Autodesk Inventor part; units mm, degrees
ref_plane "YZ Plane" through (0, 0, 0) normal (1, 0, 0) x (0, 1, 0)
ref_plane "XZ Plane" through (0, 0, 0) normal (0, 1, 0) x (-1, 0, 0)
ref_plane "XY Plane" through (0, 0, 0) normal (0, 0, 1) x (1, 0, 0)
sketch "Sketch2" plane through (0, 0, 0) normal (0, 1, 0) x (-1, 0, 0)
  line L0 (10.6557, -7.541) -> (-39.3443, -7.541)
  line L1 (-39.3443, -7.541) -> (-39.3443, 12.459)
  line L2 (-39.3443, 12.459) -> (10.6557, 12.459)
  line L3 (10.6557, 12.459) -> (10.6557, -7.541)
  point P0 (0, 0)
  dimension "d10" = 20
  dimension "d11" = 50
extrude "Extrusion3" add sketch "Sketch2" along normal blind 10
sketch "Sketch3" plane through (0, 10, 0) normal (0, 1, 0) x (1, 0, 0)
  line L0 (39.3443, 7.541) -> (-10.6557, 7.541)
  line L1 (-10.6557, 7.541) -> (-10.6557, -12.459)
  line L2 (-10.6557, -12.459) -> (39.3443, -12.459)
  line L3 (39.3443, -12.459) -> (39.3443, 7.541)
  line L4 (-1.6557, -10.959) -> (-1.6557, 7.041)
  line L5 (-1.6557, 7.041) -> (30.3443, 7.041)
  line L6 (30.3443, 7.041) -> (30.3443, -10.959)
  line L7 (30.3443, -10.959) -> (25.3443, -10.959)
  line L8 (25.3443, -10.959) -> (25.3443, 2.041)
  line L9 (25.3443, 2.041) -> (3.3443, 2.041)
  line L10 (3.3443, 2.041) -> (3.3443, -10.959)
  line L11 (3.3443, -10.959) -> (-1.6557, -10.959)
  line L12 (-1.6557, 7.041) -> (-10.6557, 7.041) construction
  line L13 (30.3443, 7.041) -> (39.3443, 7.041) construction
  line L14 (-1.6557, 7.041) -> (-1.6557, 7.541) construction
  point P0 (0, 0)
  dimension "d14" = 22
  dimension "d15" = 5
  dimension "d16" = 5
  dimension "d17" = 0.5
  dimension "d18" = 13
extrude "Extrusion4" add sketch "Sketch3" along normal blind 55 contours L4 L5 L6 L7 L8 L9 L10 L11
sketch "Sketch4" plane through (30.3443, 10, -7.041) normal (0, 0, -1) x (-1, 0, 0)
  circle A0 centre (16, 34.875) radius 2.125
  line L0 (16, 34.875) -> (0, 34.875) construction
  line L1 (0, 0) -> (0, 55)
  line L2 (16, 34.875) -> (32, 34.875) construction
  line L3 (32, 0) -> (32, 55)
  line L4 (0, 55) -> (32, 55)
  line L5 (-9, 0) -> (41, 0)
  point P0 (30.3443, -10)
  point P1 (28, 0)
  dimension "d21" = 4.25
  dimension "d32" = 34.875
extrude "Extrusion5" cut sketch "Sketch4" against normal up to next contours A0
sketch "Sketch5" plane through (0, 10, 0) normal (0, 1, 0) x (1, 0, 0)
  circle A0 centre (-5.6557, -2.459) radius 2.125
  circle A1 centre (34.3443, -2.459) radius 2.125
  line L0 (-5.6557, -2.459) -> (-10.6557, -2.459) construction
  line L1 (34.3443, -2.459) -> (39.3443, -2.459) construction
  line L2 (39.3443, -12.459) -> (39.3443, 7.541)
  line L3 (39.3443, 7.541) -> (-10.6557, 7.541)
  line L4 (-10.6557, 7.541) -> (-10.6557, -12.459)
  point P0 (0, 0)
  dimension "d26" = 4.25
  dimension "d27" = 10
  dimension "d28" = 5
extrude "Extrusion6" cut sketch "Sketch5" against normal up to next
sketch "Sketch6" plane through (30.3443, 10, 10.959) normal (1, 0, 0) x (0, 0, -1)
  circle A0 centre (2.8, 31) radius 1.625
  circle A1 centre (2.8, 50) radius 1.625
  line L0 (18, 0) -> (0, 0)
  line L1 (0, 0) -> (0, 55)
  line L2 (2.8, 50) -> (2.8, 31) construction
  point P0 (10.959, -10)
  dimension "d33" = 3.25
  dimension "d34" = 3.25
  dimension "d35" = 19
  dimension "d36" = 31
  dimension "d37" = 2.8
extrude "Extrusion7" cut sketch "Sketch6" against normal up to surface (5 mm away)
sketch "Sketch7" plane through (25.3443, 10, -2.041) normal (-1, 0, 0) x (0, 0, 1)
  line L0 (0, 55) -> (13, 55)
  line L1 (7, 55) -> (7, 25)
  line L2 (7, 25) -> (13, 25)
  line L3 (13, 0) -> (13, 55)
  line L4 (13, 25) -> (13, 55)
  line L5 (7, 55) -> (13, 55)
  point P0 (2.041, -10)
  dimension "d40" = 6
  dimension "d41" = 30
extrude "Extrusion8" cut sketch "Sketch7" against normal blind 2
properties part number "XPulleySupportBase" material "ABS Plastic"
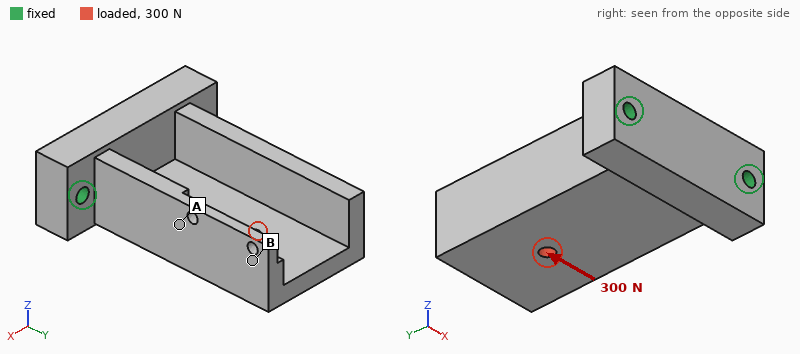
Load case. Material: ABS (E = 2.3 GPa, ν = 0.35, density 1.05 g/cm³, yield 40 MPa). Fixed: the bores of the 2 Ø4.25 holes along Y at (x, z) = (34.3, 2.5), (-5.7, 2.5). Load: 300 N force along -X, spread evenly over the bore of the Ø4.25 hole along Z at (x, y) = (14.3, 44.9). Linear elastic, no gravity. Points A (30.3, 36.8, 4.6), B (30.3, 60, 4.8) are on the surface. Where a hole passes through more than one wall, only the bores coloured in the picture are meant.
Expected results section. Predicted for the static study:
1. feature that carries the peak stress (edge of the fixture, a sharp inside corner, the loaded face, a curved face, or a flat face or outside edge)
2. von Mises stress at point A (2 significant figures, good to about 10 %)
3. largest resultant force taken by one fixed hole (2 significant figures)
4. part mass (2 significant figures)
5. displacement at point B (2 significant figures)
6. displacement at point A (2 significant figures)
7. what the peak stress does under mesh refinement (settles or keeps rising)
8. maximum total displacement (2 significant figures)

edge of the fixture
2.2 MPa
360 N
26 g
0.44 mm
0.24 mm
keeps rising
0.53 mm
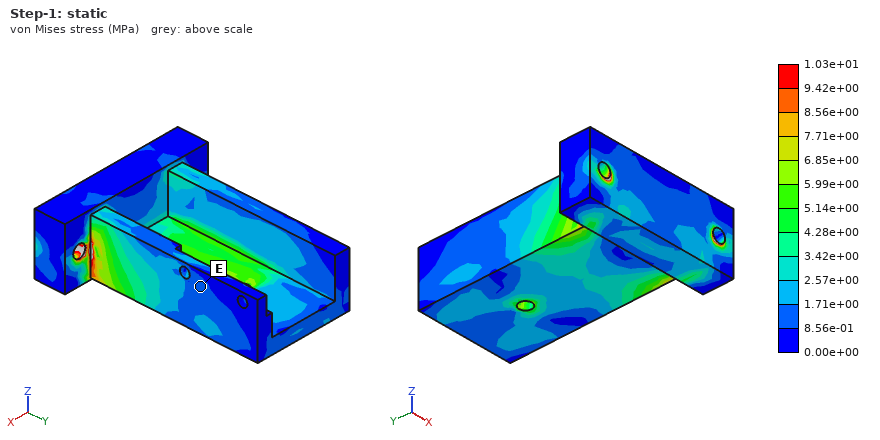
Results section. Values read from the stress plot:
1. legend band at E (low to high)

8.56e-01 to 1.71e+00 MPa
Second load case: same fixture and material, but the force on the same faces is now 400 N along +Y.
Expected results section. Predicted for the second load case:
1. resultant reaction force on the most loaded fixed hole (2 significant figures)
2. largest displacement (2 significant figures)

210 N
0.31 mm
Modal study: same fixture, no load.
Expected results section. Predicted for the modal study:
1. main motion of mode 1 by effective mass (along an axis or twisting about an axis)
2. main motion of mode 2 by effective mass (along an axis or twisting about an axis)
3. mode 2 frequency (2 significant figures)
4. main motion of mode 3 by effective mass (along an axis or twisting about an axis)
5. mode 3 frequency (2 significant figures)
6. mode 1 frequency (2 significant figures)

along Z
along X
1100 Hz
along X
2200 Hz
820 Hz
